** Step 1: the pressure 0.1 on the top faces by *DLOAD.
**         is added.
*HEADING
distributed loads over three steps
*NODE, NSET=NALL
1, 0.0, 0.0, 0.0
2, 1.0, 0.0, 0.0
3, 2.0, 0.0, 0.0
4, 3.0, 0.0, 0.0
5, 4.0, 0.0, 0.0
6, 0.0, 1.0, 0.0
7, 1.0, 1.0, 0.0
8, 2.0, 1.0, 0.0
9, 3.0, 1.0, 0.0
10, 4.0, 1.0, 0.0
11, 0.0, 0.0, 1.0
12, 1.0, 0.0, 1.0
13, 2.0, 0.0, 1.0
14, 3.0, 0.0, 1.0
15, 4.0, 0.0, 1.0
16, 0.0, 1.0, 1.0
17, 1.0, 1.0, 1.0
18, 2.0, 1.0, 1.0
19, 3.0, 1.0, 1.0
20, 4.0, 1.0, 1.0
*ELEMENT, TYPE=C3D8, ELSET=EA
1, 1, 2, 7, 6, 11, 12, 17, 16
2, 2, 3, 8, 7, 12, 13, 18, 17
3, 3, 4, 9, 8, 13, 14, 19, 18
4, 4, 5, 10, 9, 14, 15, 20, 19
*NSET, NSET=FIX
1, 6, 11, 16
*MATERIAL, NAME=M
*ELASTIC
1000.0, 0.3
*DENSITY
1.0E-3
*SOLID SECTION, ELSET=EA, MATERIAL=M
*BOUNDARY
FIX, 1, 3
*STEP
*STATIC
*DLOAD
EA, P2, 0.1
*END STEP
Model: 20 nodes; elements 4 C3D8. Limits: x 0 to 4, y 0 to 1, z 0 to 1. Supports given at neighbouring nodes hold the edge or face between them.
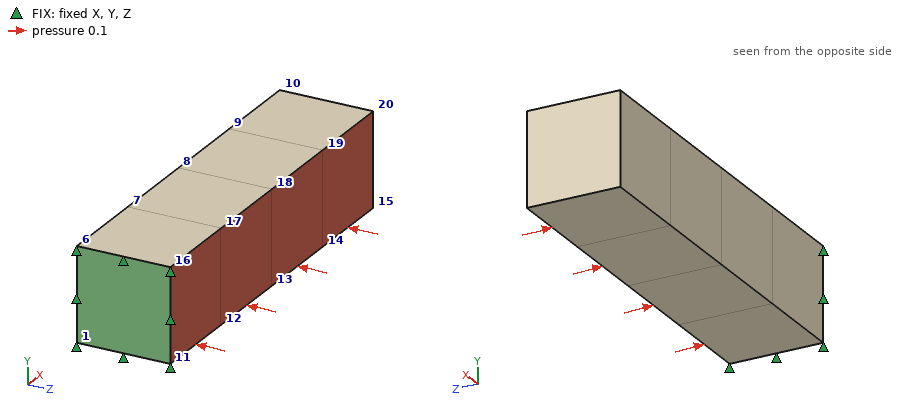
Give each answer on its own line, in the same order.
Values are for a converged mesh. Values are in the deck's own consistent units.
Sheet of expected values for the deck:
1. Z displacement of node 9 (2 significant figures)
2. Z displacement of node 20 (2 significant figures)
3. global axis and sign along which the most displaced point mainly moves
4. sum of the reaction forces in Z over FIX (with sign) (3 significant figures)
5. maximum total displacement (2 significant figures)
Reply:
-0.026
-0.038
-Z
0.400
0.039
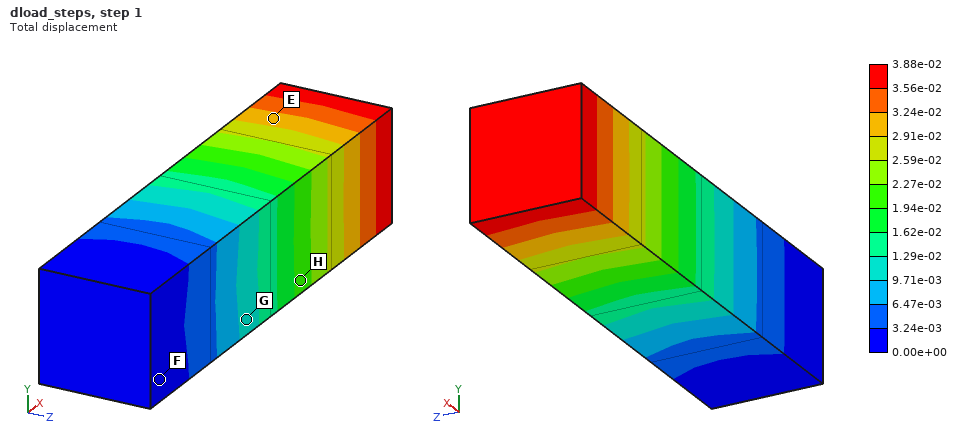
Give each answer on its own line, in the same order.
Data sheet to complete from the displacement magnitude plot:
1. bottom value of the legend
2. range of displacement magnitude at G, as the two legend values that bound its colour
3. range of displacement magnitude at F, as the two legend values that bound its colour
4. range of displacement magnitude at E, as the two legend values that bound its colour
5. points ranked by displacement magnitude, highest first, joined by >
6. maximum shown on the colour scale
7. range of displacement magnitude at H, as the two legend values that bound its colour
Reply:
0.00e+00
9.71e-03 to 1.29e-02
0.00e+00 to 3.24e-03
2.91e-02 to 3.24e-02
E > H > G > F
3.88e-02
1.94e-02 to 2.27e-02
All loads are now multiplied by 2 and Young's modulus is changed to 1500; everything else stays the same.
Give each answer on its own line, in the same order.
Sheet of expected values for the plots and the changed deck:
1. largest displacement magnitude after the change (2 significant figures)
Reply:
0.052
